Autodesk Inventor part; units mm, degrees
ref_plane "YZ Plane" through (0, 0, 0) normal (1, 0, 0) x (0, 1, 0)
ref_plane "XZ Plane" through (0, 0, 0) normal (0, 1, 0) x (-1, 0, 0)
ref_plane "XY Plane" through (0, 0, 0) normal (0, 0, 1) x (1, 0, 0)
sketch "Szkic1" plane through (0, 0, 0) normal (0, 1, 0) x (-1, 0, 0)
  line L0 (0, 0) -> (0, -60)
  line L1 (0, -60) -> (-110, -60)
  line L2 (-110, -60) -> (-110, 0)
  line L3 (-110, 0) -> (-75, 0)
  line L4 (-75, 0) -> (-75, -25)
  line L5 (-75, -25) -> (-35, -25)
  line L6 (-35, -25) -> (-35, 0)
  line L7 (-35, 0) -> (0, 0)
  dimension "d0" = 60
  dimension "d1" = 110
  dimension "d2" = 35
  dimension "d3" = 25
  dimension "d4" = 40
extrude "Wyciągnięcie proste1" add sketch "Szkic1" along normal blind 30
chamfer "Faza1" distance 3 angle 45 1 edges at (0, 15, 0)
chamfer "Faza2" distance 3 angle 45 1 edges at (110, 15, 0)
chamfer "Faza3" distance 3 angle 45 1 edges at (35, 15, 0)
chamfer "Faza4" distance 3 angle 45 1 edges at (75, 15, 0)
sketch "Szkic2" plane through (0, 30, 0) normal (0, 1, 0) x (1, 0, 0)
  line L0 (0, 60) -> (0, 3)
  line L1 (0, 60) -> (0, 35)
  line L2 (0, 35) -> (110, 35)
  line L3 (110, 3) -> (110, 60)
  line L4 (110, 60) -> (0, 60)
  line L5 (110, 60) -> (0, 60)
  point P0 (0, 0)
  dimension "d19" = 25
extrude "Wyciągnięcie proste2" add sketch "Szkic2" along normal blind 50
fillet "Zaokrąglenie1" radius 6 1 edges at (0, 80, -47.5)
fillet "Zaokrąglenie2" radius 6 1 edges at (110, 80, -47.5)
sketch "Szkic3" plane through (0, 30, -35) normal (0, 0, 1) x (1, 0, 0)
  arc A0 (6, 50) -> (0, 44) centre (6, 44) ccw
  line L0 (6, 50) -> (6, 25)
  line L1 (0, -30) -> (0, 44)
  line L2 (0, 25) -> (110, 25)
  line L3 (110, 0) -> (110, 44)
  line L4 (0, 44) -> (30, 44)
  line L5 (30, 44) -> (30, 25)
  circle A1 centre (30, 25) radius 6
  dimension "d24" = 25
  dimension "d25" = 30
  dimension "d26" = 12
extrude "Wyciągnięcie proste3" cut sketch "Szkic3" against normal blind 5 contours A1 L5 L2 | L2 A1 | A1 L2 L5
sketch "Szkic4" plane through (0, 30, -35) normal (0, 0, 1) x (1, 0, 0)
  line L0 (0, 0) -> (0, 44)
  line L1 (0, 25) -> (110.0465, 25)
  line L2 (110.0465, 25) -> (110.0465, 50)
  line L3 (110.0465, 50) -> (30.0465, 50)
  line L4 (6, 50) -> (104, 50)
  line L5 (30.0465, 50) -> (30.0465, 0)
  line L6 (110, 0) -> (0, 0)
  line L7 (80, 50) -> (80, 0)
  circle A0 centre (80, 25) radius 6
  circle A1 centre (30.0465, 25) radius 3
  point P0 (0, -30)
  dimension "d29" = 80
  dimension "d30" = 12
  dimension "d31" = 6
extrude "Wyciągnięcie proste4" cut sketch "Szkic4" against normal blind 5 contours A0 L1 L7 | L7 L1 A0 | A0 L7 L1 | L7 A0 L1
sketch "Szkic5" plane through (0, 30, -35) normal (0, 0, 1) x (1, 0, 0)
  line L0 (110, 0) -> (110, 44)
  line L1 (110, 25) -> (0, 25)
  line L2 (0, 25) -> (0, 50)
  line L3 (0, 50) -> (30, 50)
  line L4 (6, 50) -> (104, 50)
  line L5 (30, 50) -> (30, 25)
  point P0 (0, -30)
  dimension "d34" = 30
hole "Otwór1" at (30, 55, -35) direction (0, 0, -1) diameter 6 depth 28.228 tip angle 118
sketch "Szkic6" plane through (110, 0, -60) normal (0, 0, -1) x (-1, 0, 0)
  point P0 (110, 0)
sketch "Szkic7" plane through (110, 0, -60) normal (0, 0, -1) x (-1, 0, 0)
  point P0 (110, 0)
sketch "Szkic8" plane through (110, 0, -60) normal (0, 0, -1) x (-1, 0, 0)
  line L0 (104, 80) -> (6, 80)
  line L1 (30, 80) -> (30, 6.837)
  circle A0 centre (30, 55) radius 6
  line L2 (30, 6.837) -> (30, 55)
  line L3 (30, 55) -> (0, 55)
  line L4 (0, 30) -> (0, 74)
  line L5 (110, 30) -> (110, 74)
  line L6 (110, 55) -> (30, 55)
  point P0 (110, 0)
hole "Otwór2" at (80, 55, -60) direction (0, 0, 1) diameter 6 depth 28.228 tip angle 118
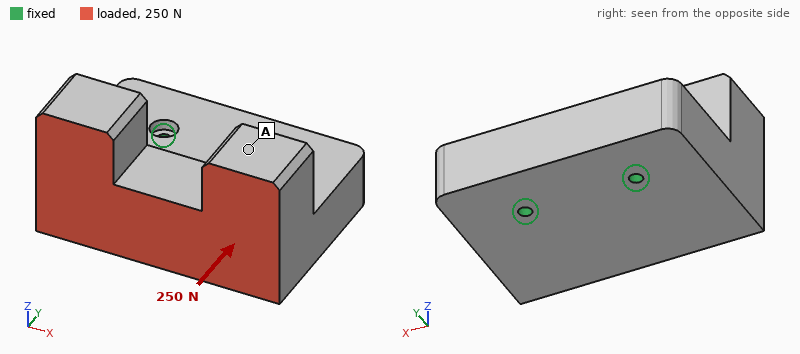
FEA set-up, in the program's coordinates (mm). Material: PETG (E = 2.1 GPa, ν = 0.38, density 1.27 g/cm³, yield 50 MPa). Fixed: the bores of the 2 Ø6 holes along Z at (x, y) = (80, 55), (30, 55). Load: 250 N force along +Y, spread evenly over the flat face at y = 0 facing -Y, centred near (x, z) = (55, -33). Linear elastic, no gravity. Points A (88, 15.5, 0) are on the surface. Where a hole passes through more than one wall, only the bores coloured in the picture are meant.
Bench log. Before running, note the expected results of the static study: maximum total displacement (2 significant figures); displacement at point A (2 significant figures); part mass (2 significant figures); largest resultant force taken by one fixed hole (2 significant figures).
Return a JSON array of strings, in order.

["56 µm", "48 µm", "380 g", "130 N"]
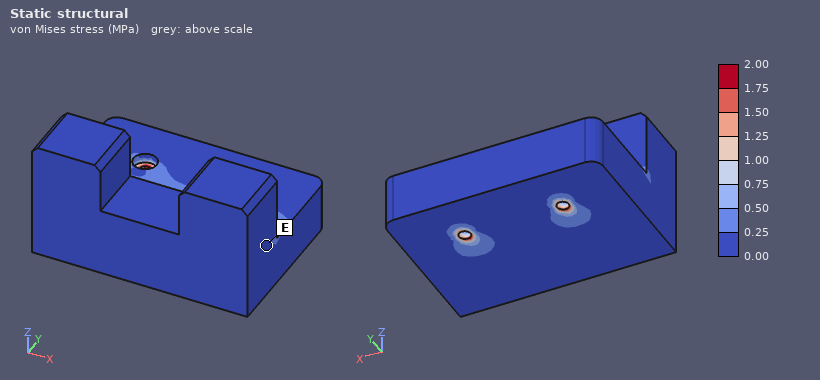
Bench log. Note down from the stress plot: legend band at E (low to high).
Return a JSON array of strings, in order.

["0.00 to 0.25 MPa"]
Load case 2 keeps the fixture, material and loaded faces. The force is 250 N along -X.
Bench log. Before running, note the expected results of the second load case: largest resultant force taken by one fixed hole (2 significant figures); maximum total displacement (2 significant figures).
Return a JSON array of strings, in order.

["300 N", "34 µm"]
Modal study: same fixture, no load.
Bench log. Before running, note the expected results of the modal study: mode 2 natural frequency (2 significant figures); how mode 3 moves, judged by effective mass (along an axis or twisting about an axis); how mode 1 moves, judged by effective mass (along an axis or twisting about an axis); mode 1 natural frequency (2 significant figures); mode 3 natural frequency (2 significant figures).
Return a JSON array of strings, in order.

["950 Hz", "along X", "along Z", "590 Hz", "1300 Hz"]
